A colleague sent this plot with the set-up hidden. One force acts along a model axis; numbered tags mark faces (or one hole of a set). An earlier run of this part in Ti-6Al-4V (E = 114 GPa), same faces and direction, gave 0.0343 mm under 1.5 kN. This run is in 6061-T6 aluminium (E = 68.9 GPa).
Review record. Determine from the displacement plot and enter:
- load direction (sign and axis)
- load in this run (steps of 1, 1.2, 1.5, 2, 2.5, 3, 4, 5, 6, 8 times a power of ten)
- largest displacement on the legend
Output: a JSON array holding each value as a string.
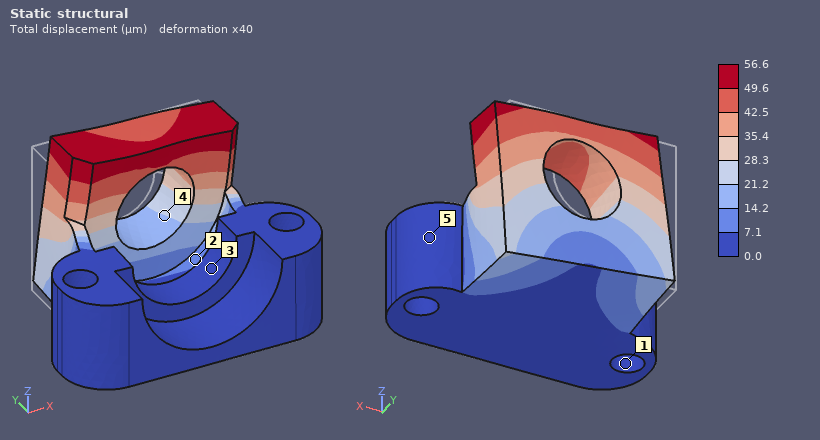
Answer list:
["+X", "1.5 kN", "56.6 µm"]
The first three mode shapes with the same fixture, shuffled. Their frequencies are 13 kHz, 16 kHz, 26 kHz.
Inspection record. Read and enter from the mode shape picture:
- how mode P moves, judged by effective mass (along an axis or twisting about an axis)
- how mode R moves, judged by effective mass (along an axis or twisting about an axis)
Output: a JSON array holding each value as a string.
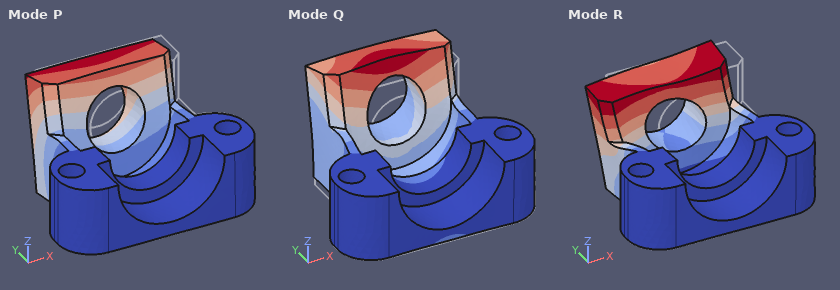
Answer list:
["along Z", "along X"]
